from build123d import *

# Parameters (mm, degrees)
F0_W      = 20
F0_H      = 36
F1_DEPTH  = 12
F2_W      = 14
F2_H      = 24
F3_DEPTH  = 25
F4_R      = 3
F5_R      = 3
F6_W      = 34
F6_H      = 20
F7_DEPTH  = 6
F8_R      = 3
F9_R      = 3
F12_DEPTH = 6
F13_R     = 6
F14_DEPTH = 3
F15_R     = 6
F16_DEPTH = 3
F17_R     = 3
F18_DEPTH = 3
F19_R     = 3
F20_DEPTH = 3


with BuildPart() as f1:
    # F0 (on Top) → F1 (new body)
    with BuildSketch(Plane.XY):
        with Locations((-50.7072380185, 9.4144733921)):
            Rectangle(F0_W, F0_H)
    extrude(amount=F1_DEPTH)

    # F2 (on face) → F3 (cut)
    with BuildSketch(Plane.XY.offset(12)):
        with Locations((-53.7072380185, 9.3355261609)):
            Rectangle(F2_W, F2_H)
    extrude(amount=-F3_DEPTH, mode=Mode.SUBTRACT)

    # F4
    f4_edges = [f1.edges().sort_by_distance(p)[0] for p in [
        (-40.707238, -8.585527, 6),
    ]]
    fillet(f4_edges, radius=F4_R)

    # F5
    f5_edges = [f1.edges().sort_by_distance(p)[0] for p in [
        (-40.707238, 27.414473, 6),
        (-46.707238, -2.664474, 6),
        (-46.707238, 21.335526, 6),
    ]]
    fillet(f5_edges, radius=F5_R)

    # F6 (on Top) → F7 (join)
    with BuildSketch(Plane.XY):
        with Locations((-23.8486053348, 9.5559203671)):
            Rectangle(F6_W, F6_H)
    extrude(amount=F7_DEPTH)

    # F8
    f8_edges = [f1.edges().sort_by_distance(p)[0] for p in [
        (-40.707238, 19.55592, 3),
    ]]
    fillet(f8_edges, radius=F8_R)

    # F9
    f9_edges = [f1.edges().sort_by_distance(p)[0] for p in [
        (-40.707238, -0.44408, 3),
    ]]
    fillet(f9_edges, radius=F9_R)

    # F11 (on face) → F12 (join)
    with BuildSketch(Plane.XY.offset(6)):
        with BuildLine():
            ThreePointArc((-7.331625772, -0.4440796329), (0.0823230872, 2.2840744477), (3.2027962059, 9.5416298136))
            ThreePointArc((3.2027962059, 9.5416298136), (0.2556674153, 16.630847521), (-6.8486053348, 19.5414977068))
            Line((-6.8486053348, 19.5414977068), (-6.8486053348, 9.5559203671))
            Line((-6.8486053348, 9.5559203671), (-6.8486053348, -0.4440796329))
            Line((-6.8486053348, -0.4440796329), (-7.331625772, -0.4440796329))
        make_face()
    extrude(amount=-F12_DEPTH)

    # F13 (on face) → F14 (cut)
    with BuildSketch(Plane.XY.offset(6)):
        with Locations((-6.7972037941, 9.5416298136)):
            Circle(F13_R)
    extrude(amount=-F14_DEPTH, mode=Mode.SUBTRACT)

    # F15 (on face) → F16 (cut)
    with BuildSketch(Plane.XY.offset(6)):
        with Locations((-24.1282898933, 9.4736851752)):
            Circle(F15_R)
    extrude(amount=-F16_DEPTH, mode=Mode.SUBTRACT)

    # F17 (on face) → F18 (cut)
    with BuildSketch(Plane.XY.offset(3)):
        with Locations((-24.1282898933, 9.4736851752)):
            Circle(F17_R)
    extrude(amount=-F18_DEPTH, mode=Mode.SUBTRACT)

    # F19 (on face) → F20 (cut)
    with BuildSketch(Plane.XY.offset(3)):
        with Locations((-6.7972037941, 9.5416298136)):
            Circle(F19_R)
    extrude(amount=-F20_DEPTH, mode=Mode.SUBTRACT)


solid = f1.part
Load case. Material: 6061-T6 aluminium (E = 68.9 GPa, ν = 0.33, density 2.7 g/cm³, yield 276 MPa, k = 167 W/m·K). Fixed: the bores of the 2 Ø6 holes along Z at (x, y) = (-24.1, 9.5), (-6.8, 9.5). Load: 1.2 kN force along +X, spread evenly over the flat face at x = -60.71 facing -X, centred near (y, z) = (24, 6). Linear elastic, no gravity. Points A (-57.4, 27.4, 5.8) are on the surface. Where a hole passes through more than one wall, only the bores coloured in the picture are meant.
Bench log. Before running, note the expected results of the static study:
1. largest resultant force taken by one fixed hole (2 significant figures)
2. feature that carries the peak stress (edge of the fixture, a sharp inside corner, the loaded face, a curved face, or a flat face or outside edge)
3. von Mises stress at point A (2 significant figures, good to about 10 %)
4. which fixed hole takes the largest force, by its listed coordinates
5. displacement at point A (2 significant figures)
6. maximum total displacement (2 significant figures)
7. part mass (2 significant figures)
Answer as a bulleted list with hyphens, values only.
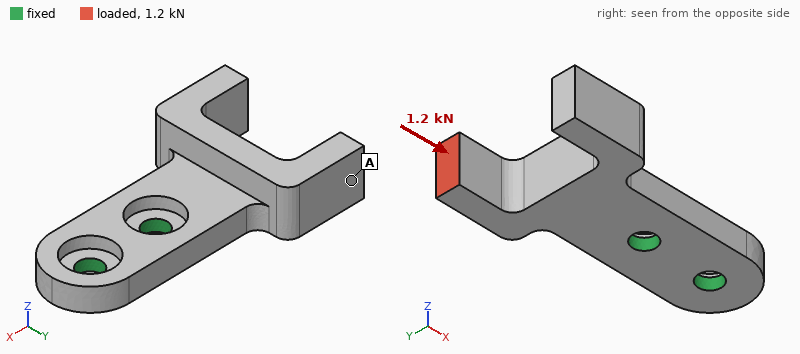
- 950 N
- a sharp inside corner
- 17 MPa
- (-24.1, 9.5)
- 0.18 mm
- 0.22 mm
- 24 g
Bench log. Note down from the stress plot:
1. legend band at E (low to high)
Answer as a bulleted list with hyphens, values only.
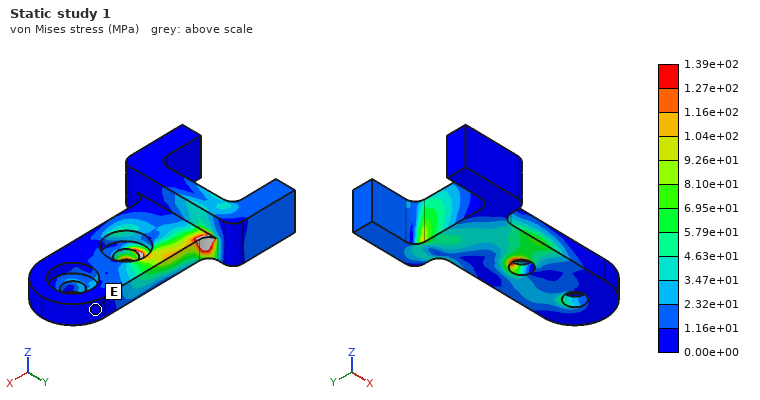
- 0.00e+00 to 1.16e+01 MPa
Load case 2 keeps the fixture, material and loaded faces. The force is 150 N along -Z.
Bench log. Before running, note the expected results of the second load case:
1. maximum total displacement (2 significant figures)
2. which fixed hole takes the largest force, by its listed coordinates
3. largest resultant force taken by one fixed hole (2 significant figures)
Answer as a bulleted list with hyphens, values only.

- 0.20 mm
- (-24.1, 9.5)
- 430 N
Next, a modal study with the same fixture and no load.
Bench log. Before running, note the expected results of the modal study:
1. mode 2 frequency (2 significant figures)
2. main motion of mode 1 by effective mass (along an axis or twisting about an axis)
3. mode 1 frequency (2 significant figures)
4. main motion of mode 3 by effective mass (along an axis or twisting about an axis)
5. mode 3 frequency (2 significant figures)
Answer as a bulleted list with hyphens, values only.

- 3400 Hz
- along Z
- 2300 Hz
- along Y
- 5100 Hz
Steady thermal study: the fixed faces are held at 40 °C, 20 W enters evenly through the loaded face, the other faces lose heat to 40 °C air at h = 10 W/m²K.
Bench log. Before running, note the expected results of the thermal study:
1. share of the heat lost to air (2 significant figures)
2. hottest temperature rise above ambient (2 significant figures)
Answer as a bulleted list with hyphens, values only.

- 3.5 %
- 59 K
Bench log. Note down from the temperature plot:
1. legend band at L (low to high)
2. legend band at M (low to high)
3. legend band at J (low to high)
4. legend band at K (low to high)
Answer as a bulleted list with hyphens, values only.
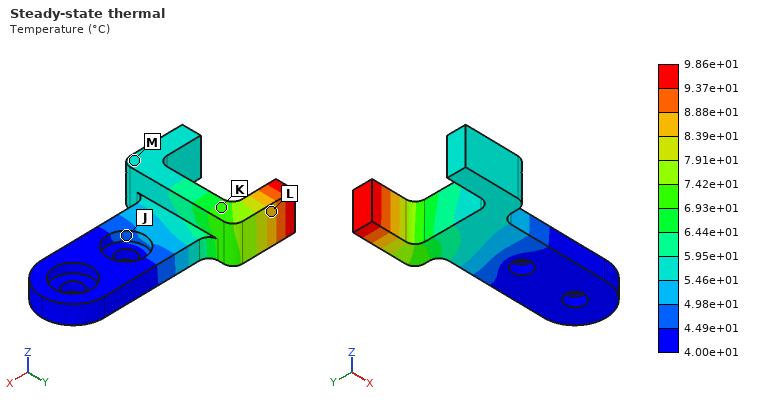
- 8.39e+01 to 8.88e+01 °C
- 5.46e+01 to 5.95e+01 °C
- 4.49e+01 to 4.98e+01 °C
- 6.93e+01 to 7.42e+01 °C
